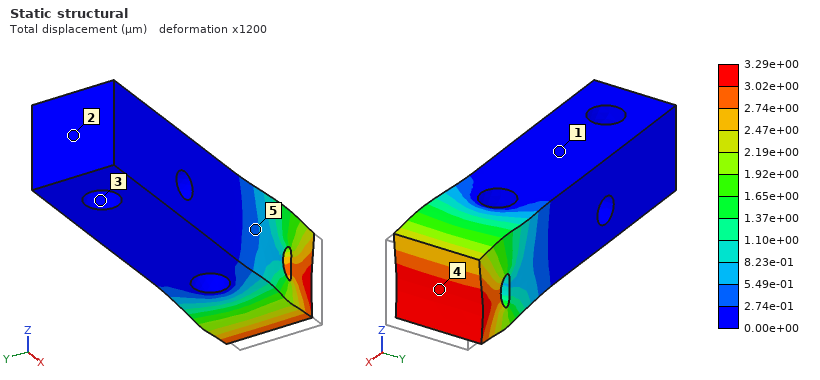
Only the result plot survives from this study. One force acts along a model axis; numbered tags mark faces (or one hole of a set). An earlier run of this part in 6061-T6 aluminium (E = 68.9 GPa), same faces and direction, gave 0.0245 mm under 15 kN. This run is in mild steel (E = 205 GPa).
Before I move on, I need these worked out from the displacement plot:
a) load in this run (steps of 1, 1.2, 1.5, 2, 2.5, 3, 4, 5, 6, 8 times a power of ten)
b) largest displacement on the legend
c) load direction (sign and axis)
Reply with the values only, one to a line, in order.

6 kN
3.29e+00 µm
-X
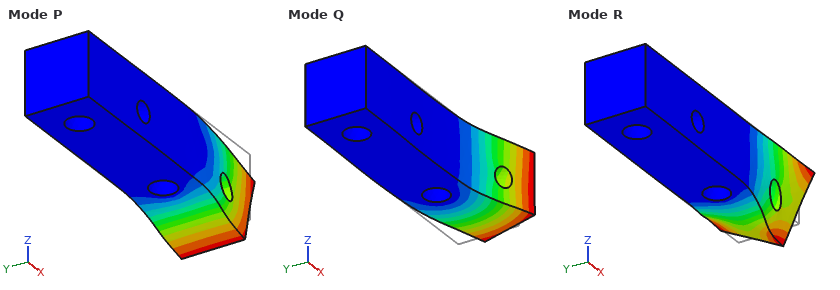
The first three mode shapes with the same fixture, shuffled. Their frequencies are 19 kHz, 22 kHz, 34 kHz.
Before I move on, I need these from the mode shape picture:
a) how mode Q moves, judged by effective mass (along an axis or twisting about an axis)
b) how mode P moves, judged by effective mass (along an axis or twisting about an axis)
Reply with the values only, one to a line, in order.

along Y
along Z
